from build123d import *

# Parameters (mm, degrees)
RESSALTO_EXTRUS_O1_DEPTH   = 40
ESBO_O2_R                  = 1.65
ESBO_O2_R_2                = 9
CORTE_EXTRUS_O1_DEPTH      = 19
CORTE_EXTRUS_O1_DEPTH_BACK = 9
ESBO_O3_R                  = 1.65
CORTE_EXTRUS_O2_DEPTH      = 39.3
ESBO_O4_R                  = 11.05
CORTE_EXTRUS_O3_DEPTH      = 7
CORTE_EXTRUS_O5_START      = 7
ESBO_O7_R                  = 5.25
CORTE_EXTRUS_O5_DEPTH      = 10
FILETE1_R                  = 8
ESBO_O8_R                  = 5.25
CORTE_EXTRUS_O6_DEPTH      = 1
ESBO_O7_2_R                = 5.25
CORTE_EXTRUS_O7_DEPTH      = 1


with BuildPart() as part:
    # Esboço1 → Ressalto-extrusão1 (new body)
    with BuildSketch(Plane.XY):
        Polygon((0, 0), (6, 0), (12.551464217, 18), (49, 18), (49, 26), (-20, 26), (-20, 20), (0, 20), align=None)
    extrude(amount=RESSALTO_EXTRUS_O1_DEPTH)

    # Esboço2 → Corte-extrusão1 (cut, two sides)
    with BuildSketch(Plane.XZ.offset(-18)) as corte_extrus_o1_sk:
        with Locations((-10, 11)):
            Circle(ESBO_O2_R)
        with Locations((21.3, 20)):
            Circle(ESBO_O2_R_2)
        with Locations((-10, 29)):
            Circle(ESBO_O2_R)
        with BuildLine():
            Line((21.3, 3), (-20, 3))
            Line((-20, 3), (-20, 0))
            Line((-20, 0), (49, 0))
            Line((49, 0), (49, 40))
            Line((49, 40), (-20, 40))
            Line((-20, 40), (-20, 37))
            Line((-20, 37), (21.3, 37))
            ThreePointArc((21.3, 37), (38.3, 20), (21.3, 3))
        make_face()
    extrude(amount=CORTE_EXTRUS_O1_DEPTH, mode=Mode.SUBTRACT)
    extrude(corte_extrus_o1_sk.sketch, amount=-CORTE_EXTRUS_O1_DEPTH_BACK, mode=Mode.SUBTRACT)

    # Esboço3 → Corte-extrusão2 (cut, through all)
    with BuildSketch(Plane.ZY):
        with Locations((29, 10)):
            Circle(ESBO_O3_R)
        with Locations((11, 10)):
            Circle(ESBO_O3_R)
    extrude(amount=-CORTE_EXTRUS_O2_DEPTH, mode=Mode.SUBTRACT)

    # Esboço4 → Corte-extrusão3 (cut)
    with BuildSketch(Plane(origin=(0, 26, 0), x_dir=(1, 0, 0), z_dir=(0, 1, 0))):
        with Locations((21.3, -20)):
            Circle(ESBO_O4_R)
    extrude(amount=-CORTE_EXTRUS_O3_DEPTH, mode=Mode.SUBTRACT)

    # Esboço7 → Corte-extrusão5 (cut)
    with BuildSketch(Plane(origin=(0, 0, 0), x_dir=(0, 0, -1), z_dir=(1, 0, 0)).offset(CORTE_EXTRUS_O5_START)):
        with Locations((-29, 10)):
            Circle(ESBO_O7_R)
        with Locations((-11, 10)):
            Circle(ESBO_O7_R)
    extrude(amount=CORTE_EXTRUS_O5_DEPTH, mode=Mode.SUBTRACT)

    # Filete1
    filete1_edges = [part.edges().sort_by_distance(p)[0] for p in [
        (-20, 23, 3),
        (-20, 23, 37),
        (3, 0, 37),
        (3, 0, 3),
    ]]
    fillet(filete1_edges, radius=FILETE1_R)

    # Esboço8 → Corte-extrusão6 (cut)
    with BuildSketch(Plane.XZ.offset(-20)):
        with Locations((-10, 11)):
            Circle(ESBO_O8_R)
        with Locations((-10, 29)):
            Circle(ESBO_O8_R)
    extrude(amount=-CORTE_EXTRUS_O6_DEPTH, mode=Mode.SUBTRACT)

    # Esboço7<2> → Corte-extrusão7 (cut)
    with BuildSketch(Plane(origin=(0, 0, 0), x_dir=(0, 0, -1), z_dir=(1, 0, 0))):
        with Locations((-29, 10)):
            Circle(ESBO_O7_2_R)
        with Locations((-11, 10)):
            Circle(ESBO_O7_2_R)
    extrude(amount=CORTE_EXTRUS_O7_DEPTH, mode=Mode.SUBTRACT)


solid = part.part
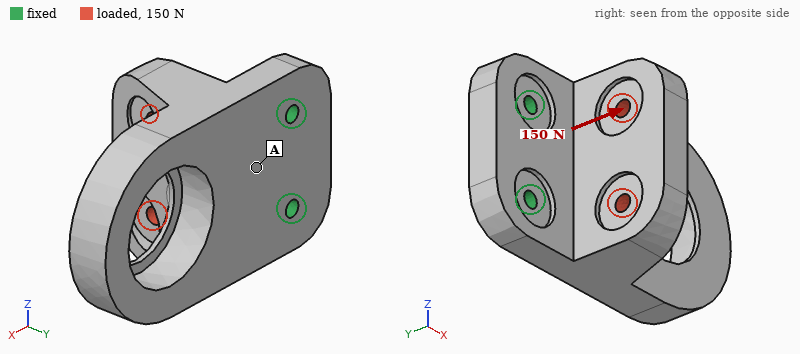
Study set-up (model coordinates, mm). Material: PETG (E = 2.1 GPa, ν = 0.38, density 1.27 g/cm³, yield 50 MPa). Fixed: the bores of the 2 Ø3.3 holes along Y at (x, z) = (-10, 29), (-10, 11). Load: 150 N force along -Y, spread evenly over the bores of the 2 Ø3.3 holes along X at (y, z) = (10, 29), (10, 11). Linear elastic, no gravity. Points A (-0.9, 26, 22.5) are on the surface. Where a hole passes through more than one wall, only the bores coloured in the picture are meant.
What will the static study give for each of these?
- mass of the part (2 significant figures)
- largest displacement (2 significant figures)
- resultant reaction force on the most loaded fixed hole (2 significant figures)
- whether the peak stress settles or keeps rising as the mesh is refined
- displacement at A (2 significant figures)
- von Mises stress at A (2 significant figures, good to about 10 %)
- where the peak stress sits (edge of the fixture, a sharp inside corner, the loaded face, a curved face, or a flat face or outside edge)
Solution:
19 g
0.74 mm
75 N
keeps rising
0.11 mm
3.2 MPa
edge of the fixture
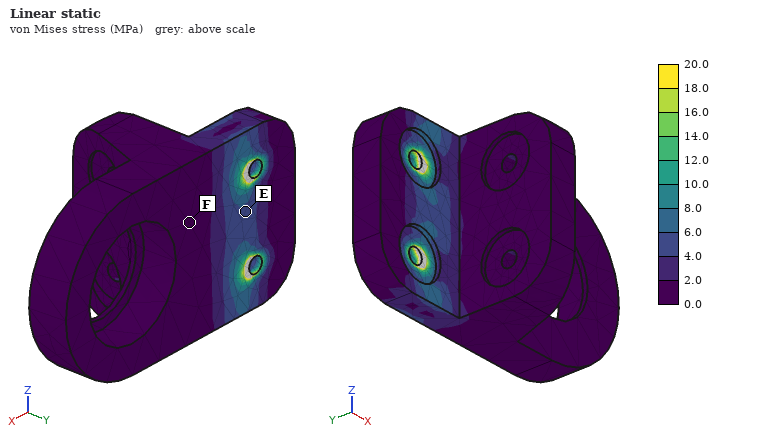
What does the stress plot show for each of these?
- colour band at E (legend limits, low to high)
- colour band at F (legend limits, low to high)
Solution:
4.0 to 6.0 MPa
0.0 to 2.0 MPa
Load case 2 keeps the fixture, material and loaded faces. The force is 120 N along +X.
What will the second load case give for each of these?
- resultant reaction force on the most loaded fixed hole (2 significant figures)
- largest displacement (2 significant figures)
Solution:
61 N
0.84 mm
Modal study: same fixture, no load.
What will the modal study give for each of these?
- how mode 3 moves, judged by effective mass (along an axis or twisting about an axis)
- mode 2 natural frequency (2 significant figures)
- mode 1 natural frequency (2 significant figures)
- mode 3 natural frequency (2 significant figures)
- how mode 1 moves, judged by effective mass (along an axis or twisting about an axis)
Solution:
along Z
1600 Hz
540 Hz
1900 Hz
along Y
